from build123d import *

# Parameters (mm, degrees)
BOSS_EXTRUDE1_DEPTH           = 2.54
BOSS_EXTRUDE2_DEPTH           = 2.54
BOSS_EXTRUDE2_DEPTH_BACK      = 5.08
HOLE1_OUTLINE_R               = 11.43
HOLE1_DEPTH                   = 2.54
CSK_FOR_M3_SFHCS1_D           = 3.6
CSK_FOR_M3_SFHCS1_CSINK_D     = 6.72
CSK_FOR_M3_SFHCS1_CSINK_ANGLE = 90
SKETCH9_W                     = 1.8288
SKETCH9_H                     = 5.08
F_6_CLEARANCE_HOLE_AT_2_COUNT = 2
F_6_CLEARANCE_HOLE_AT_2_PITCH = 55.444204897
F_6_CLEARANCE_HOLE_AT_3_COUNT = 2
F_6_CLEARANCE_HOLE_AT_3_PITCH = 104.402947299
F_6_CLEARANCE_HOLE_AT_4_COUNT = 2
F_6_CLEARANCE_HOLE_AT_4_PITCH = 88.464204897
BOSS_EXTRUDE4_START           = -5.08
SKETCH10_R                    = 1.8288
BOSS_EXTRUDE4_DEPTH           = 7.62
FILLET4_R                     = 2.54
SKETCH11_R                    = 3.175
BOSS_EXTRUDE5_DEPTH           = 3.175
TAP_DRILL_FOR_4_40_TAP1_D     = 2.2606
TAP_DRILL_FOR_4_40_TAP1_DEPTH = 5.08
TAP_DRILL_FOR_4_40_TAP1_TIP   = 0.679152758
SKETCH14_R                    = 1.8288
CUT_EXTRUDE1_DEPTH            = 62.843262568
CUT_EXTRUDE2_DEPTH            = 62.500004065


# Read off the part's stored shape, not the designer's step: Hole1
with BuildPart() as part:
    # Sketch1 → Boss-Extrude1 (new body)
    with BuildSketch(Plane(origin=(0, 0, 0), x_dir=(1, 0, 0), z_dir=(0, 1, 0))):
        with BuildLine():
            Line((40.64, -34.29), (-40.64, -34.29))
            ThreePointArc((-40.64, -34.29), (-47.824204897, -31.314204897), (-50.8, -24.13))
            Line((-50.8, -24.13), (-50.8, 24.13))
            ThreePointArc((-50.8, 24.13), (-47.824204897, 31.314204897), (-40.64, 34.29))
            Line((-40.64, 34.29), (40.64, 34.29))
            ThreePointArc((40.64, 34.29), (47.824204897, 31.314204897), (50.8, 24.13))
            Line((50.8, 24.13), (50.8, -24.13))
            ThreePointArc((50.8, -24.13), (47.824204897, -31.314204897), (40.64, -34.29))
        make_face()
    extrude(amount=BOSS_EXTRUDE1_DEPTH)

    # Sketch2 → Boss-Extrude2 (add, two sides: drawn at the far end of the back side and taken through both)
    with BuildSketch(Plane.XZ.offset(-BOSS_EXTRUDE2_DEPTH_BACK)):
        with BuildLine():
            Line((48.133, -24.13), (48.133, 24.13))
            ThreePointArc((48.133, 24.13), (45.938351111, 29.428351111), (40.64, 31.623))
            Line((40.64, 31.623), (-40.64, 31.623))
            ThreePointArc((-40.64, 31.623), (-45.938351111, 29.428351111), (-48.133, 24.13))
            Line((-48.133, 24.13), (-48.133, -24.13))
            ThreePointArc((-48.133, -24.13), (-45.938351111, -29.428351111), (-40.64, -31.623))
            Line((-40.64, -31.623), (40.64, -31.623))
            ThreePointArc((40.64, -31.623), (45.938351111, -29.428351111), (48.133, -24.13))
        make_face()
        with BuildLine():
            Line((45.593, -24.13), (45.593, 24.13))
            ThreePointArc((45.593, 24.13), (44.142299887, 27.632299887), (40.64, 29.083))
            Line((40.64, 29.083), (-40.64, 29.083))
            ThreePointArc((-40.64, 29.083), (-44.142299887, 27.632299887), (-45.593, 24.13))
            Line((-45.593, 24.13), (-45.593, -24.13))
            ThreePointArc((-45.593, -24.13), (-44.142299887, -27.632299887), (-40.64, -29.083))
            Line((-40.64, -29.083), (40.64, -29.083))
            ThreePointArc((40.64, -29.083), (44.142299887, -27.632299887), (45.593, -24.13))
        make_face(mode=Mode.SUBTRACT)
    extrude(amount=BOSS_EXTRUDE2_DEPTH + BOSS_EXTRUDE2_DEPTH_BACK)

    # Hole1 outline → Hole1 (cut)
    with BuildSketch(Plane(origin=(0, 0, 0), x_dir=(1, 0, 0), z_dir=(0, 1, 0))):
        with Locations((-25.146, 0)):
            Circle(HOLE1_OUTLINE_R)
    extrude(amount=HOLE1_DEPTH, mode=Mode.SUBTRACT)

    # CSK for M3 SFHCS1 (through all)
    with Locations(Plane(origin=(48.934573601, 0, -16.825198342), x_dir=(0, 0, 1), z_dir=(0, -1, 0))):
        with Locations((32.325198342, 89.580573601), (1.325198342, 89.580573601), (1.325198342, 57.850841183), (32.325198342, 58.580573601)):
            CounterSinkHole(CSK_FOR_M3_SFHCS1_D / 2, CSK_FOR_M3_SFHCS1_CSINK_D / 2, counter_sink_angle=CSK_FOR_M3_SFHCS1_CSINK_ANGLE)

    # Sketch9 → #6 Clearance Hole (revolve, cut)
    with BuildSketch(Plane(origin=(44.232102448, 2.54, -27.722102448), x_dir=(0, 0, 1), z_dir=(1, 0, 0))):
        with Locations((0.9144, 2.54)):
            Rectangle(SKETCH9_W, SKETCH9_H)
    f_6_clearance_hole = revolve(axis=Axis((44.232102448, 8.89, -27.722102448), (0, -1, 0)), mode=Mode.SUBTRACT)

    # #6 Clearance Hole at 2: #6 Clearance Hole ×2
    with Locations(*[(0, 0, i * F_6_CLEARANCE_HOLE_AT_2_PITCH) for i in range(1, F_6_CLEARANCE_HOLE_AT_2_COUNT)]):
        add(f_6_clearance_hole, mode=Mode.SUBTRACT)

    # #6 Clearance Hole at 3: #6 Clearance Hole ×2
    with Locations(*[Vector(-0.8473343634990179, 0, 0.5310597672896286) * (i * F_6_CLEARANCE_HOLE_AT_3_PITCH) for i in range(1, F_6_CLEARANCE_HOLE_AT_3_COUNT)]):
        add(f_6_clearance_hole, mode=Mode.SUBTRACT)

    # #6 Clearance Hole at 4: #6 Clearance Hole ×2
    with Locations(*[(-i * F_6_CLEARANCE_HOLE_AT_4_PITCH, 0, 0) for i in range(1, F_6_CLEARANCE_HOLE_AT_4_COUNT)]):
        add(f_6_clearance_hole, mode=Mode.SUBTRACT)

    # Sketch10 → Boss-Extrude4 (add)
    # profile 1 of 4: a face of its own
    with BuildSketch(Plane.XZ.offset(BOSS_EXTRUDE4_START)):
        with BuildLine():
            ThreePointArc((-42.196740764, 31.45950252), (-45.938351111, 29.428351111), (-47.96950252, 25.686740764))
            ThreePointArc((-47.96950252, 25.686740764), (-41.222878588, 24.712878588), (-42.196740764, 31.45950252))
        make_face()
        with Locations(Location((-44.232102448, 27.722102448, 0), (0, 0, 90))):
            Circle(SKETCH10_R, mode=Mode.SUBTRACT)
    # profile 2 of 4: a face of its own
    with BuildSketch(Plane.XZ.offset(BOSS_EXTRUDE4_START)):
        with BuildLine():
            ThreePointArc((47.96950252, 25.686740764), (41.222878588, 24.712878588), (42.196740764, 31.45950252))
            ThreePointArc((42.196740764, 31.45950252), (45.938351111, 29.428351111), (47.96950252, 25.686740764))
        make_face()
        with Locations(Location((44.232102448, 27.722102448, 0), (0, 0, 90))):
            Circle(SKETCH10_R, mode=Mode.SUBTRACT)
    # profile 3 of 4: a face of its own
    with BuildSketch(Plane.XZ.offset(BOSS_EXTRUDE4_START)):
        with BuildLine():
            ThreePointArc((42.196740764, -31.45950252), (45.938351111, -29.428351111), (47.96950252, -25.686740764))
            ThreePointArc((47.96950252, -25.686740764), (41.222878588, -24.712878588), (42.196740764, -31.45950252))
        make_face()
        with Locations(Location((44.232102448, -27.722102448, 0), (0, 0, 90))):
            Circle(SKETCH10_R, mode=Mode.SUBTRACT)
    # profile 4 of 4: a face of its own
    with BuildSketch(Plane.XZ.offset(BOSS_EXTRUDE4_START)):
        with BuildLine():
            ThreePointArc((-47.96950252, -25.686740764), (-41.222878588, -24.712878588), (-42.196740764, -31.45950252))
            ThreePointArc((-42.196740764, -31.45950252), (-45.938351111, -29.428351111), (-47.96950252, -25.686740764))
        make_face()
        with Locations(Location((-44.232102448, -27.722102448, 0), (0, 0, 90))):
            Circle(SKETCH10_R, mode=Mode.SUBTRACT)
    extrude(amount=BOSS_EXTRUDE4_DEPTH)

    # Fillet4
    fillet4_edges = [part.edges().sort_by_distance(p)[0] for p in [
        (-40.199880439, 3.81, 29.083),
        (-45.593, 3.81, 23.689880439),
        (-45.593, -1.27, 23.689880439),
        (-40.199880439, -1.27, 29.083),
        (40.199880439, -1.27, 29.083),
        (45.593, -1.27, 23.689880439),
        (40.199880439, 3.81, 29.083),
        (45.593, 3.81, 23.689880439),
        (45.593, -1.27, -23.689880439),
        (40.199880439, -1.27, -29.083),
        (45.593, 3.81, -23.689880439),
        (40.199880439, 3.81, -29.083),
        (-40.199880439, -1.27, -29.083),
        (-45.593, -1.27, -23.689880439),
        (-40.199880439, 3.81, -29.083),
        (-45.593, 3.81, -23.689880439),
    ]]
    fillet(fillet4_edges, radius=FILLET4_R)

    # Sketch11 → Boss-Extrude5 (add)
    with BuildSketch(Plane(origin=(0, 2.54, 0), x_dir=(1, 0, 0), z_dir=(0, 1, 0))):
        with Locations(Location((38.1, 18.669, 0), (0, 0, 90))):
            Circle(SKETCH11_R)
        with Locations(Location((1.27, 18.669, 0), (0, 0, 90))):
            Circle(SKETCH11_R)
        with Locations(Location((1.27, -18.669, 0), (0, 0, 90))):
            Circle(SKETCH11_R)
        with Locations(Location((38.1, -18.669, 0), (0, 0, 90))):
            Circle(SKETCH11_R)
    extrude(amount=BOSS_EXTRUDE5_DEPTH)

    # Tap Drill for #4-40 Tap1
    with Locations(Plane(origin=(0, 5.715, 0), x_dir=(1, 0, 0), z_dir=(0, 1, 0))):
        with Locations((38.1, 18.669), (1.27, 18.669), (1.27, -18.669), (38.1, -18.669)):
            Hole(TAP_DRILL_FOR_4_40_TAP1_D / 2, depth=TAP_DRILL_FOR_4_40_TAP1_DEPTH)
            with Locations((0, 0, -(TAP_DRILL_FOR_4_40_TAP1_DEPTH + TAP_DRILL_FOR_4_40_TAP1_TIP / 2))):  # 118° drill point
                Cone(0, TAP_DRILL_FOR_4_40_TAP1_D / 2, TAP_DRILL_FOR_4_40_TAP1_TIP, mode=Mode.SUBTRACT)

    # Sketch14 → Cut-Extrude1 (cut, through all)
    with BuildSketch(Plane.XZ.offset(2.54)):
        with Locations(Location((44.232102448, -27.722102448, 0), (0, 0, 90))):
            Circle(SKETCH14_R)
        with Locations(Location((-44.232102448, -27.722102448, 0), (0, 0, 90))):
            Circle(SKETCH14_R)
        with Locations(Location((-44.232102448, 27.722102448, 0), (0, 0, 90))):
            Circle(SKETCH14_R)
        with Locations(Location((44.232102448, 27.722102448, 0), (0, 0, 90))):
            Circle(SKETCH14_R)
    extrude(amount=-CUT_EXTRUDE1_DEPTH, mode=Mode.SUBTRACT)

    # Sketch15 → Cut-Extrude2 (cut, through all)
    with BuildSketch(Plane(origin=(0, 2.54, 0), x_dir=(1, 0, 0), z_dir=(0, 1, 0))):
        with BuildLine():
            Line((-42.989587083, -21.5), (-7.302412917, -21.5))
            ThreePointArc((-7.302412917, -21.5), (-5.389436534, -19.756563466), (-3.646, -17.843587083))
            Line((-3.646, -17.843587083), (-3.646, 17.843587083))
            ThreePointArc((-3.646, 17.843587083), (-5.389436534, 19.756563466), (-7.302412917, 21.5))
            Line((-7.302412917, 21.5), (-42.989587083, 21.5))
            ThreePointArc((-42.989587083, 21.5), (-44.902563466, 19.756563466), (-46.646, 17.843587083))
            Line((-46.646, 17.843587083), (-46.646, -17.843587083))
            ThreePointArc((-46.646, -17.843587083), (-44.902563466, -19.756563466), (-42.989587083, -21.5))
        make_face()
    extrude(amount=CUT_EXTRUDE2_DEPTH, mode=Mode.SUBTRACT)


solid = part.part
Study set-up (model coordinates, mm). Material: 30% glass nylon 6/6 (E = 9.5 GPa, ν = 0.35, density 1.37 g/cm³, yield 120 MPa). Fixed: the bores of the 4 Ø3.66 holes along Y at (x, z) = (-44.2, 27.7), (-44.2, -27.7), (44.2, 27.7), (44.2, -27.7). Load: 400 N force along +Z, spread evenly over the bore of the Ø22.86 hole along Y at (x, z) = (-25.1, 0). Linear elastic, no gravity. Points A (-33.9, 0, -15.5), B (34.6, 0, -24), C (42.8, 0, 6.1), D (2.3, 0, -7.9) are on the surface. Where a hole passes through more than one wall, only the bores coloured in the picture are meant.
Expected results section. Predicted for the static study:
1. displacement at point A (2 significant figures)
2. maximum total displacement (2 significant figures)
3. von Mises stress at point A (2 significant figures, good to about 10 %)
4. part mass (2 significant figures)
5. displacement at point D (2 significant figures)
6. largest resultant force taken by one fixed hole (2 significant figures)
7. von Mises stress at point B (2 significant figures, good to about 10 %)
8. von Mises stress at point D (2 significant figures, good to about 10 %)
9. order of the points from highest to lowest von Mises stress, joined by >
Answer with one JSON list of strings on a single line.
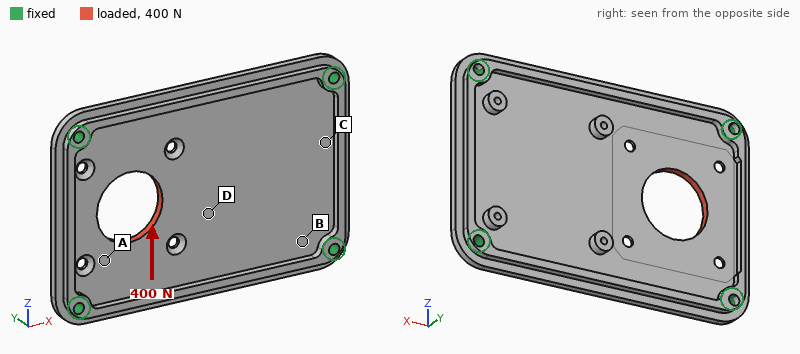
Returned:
["8.5 µm", "18 µm", "3.3 MPa", "28 g", "11 µm", "150 N", "1.7 MPa", "1.1 MPa", "A > B > D > C"]
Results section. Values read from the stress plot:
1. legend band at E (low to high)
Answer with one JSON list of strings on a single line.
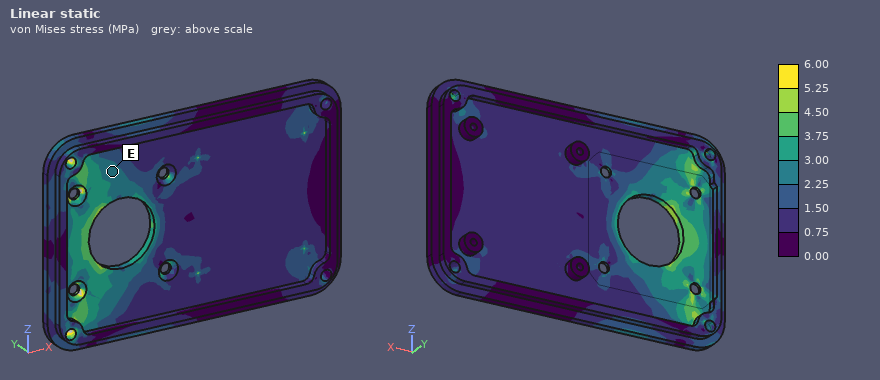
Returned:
["2.25 to 3.00 MPa"]
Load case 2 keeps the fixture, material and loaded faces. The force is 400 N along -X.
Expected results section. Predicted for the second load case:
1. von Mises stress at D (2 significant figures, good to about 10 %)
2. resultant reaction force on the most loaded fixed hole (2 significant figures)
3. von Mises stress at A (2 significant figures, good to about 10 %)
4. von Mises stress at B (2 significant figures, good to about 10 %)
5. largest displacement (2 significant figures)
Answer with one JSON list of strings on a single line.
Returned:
["1.6 MPa", "130 N", "2.9 MPa", "1.4 MPa", "18 µm"]
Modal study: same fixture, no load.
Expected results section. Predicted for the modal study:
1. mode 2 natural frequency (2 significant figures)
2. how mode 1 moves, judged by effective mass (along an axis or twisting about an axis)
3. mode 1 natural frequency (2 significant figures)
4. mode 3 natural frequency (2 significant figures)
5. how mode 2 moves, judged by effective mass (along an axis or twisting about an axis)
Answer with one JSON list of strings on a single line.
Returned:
["1900 Hz", "along Y", "1200 Hz", "2600 Hz", "twisting about X"]
